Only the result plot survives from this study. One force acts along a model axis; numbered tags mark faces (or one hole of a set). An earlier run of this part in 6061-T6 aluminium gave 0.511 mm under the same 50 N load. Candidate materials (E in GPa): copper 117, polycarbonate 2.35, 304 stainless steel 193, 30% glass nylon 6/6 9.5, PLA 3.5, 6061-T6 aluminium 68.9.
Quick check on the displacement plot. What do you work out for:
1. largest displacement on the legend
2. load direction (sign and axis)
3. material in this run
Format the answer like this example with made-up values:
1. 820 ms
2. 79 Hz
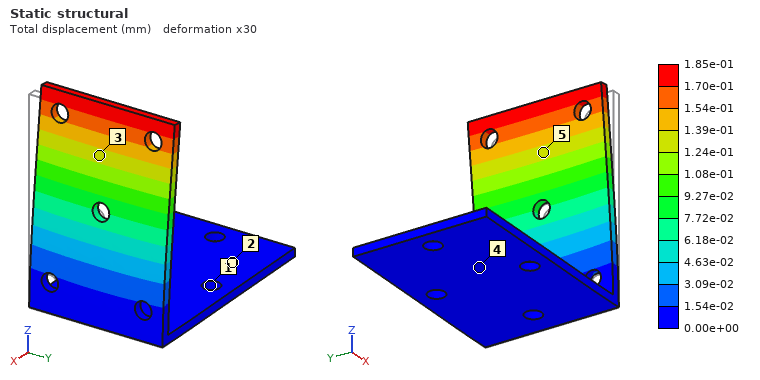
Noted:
1. 1.85e-01 mm
2. -X
3. 304 stainless steel
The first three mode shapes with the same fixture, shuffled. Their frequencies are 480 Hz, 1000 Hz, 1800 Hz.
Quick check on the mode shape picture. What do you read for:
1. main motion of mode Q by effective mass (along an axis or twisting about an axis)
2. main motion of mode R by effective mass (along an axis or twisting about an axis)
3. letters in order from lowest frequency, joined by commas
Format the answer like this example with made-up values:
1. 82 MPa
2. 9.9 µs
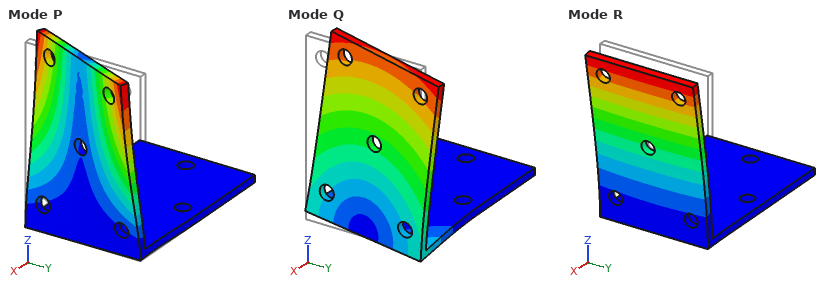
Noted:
1. along Y
2. along X
3. R, Q, P
